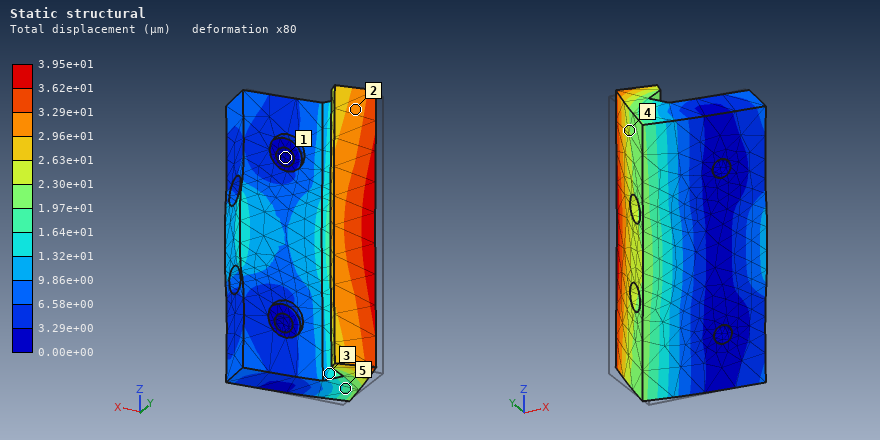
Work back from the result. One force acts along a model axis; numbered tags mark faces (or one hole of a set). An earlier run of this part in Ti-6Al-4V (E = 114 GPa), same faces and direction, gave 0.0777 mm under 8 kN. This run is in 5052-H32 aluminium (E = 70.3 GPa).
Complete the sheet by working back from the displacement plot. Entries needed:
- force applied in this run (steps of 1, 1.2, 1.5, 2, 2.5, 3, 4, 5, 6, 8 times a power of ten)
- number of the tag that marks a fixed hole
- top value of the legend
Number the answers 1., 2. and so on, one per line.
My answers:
1. 2.5 kN
2. 1
3. 3.95e+01 µm
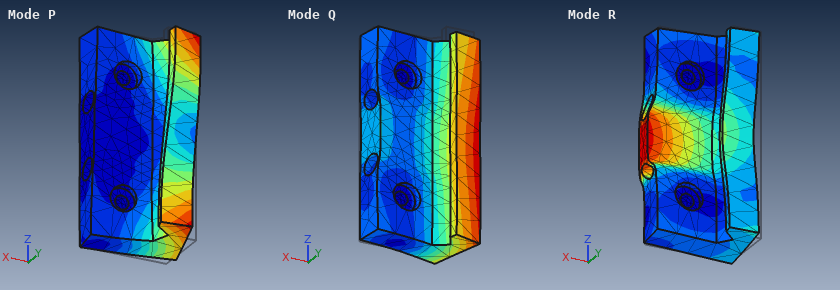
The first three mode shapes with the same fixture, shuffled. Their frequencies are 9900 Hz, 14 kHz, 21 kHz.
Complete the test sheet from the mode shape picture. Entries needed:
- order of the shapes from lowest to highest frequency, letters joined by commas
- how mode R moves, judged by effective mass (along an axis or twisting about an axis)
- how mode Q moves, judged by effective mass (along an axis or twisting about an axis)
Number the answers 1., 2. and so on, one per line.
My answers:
1. Q, P, R
2. along Y
3. along Y
